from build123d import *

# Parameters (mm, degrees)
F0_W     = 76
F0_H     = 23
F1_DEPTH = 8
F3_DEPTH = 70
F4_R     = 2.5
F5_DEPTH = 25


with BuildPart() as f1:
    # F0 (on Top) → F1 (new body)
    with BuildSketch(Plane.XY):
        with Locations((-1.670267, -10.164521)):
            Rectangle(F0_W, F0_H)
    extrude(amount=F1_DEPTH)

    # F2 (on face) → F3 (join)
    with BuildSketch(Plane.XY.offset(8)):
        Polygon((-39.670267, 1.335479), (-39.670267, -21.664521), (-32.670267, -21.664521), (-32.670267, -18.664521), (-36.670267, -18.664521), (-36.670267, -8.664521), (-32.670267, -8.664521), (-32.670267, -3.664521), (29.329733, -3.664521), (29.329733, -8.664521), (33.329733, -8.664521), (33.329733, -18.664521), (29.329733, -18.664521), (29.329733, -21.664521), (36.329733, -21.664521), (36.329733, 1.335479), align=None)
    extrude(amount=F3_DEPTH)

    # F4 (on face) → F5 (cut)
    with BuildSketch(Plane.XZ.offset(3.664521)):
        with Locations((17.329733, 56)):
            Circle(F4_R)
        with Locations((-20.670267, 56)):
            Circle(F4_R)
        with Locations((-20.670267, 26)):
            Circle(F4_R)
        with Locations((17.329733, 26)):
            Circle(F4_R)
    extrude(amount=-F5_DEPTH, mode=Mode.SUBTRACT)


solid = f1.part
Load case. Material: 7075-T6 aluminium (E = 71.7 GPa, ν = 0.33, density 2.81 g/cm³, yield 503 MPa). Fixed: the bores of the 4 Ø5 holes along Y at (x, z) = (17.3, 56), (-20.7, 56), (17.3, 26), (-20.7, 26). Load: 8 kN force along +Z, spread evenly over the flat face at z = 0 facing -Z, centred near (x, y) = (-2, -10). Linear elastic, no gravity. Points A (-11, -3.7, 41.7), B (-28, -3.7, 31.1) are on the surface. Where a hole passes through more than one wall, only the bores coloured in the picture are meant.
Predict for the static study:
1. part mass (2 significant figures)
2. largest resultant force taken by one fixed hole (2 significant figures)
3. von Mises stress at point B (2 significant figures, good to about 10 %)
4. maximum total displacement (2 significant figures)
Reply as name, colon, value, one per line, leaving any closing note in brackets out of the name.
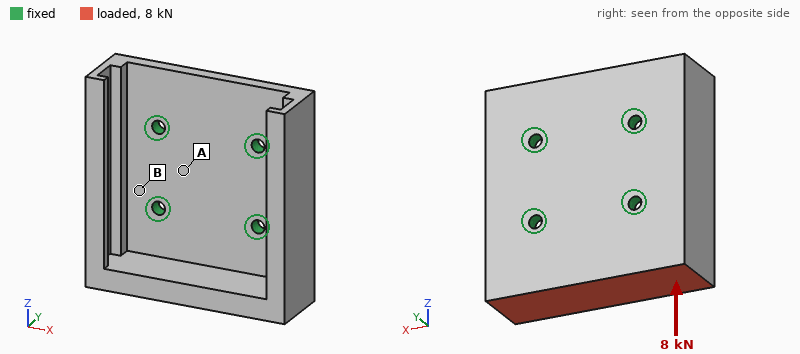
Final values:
part mass: 150 g
largest resultant force taken by one fixed hole: 3.0 kN
von Mises stress at point B: 45 MPa
maximum total displacement: 0.17 mm
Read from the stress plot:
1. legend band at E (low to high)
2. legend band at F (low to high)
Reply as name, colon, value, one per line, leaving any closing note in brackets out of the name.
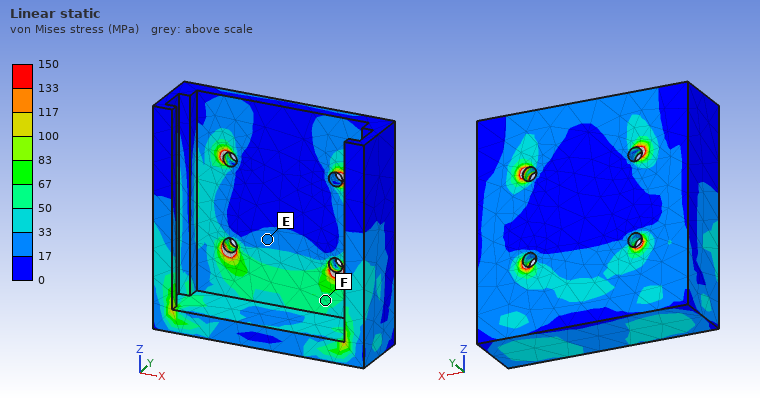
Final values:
legend band at E: 17 to 33 MPa
legend band at F: 50 to 67 MPa
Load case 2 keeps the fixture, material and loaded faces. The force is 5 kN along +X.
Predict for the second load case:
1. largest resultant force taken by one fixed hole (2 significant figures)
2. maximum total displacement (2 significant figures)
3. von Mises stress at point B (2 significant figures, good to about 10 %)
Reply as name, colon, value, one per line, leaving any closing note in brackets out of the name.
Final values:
largest resultant force taken by one fixed hole: 3.5 kN
maximum total displacement: 85 µm
von Mises stress at point B: 27 MPa
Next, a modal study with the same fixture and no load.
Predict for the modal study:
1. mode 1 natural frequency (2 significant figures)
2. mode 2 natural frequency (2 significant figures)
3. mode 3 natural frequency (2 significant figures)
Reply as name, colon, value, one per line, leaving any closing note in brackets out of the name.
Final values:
mode 1 natural frequency: 3700 Hz
mode 2 natural frequency: 4000 Hz
mode 3 natural frequency: 4600 Hz
